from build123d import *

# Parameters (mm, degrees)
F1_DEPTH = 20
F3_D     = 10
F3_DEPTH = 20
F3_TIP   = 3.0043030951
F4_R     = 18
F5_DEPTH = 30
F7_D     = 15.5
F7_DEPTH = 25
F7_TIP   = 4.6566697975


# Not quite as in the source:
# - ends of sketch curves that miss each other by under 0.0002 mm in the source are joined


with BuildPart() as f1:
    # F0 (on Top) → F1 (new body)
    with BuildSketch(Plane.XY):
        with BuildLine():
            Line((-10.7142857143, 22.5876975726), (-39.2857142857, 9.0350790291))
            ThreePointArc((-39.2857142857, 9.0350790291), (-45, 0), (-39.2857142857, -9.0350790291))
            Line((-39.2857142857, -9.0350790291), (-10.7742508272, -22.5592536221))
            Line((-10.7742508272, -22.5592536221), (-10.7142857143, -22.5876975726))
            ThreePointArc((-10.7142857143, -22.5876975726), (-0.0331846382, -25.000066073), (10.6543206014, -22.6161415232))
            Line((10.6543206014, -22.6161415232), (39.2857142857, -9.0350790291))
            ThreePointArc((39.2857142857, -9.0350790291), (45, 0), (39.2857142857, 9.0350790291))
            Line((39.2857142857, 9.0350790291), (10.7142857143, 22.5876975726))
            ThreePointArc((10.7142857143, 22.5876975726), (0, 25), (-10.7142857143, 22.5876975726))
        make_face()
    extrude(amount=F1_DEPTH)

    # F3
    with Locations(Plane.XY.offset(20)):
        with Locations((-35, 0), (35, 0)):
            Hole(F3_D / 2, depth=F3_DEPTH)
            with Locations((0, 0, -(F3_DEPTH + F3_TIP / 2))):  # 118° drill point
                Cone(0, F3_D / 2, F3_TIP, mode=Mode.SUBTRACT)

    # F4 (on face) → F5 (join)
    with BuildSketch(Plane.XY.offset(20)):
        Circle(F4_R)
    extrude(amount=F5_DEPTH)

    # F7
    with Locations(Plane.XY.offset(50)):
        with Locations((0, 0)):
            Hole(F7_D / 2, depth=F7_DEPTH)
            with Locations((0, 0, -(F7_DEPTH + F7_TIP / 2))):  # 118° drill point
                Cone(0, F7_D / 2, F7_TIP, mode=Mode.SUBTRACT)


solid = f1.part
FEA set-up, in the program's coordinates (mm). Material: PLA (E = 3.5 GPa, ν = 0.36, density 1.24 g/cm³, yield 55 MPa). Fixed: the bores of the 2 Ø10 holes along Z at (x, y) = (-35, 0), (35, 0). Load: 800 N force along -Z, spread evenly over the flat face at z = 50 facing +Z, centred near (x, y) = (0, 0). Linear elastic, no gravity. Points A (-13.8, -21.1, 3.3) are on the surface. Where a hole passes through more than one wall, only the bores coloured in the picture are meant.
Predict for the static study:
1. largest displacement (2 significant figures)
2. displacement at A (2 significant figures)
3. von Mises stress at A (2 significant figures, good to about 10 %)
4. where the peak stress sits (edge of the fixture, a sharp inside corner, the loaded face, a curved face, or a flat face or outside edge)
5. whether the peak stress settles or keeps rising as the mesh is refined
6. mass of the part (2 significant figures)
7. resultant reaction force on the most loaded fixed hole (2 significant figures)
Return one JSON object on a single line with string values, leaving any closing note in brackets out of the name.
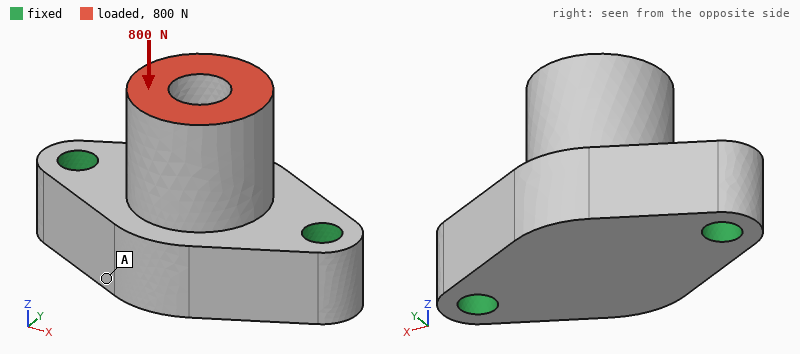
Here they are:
{"largest displacement": "27 µm", "displacement at A": "19 µm", "von Mises stress at A": "0.58 MPa", "where the peak stress sits": "edge of the fixture", "whether the peak stress settles or keeps rising as the mesh is refined": "keeps rising", "mass of the part": "100 g", "resultant reaction force on the most loaded fixed hole": "410 N"}
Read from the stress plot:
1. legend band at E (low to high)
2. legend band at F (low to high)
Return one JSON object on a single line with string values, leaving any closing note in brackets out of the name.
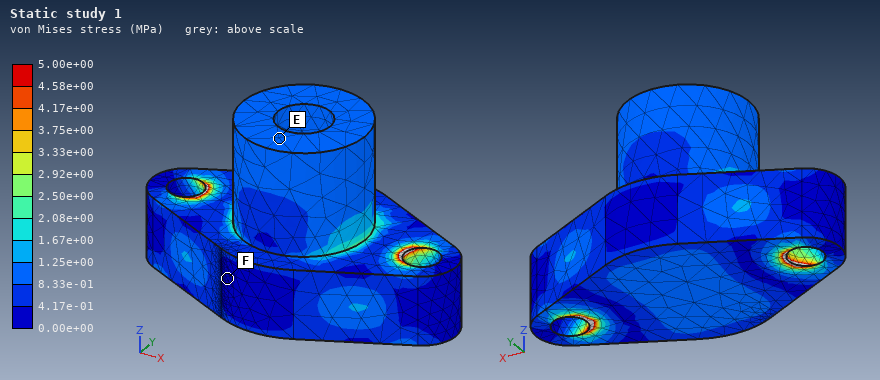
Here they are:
{"legend band at E": "8.33e-01 to 1.25e+00 MPa", "legend band at F": "0.00e+00 to 4.17e-01 MPa"}
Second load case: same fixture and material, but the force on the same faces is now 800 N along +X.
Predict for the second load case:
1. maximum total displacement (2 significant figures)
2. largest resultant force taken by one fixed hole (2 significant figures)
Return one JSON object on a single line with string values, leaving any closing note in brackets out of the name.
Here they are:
{"maximum total displacement": "0.12 mm", "largest resultant force taken by one fixed hole": "690 N"}
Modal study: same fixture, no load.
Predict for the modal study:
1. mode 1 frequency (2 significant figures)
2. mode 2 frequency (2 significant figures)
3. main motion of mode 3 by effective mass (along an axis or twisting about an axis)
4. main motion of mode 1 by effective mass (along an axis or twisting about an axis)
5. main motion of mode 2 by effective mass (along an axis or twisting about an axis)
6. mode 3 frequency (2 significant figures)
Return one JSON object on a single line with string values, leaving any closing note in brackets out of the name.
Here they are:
{"mode 1 frequency": "2000 Hz", "mode 2 frequency": "3600 Hz", "main motion of mode 3 by effective mass": "along X", "main motion of mode 1 by effective mass": "along Y", "main motion of mode 2 by effective mass": "along Z", "mode 3 frequency": "3800 Hz"}
